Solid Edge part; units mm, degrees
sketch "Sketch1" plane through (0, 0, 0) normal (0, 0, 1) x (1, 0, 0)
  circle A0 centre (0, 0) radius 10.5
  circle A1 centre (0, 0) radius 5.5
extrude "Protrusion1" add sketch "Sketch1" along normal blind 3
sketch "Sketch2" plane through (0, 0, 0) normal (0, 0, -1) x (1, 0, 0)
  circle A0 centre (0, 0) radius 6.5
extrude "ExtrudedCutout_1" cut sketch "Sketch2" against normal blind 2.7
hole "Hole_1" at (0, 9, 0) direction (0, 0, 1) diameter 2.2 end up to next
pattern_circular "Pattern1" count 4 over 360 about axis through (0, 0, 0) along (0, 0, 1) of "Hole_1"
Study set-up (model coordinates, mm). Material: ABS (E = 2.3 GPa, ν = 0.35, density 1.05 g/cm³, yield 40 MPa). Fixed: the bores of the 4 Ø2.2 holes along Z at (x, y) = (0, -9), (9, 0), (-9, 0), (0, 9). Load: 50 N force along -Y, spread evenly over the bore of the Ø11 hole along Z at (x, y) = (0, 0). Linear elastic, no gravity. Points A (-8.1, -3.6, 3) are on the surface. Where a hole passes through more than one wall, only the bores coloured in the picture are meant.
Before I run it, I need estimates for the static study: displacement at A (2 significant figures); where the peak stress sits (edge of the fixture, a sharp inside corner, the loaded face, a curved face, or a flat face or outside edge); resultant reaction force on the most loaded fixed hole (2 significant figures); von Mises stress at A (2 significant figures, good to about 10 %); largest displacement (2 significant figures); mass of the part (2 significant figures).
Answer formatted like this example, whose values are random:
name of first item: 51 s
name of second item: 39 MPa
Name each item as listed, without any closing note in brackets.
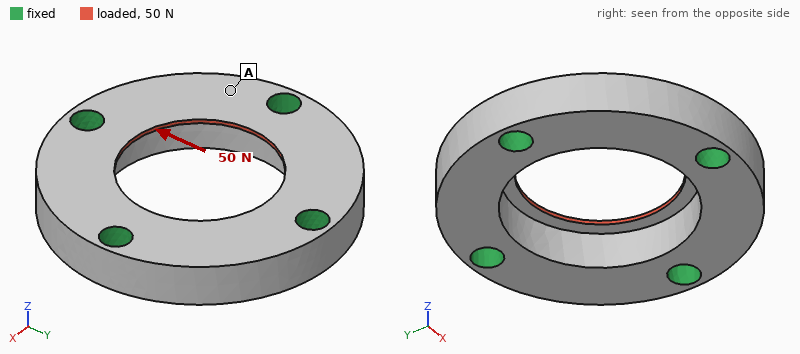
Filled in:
displacement at A: 2.5 µm
where the peak stress sits: a sharp inside corner
resultant reaction force on the most loaded fixed hole: 14 N
von Mises stress at A: 1.1 MPa
largest displacement: 9.9 µm
mass of the part: 0.64 g
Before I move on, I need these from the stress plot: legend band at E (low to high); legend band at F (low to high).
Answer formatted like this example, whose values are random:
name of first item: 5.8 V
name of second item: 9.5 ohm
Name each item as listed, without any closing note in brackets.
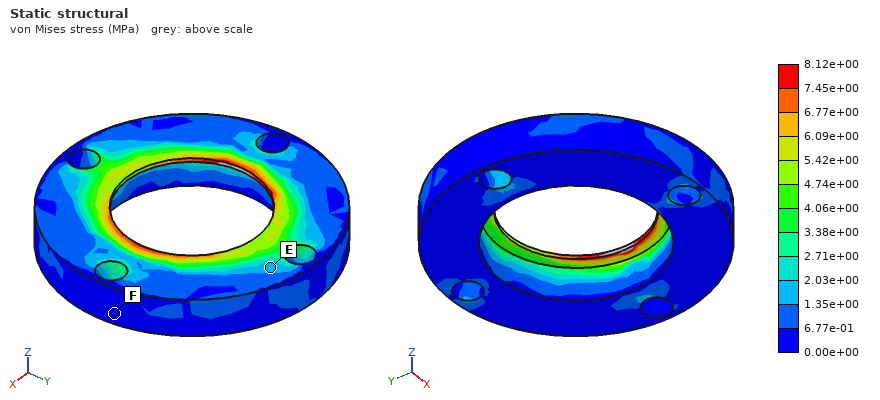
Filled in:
legend band at E: 1.35e+00 to 2.03e+00 MPa
legend band at F: 0.00e+00 to 6.77e-01 MPa
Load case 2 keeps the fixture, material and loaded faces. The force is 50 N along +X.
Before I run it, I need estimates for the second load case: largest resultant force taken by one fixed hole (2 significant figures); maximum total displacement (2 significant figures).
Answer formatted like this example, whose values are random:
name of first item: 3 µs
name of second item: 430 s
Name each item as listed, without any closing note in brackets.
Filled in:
largest resultant force taken by one fixed hole: 14 N
maximum total displacement: 9.9 µm
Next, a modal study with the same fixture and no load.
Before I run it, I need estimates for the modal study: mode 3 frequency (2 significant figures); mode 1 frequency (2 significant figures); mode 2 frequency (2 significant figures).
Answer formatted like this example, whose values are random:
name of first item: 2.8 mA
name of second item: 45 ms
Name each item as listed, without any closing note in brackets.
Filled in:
mode 3 frequency: 21 kHz
mode 1 frequency: 21 kHz
mode 2 frequency: 21 kHz
